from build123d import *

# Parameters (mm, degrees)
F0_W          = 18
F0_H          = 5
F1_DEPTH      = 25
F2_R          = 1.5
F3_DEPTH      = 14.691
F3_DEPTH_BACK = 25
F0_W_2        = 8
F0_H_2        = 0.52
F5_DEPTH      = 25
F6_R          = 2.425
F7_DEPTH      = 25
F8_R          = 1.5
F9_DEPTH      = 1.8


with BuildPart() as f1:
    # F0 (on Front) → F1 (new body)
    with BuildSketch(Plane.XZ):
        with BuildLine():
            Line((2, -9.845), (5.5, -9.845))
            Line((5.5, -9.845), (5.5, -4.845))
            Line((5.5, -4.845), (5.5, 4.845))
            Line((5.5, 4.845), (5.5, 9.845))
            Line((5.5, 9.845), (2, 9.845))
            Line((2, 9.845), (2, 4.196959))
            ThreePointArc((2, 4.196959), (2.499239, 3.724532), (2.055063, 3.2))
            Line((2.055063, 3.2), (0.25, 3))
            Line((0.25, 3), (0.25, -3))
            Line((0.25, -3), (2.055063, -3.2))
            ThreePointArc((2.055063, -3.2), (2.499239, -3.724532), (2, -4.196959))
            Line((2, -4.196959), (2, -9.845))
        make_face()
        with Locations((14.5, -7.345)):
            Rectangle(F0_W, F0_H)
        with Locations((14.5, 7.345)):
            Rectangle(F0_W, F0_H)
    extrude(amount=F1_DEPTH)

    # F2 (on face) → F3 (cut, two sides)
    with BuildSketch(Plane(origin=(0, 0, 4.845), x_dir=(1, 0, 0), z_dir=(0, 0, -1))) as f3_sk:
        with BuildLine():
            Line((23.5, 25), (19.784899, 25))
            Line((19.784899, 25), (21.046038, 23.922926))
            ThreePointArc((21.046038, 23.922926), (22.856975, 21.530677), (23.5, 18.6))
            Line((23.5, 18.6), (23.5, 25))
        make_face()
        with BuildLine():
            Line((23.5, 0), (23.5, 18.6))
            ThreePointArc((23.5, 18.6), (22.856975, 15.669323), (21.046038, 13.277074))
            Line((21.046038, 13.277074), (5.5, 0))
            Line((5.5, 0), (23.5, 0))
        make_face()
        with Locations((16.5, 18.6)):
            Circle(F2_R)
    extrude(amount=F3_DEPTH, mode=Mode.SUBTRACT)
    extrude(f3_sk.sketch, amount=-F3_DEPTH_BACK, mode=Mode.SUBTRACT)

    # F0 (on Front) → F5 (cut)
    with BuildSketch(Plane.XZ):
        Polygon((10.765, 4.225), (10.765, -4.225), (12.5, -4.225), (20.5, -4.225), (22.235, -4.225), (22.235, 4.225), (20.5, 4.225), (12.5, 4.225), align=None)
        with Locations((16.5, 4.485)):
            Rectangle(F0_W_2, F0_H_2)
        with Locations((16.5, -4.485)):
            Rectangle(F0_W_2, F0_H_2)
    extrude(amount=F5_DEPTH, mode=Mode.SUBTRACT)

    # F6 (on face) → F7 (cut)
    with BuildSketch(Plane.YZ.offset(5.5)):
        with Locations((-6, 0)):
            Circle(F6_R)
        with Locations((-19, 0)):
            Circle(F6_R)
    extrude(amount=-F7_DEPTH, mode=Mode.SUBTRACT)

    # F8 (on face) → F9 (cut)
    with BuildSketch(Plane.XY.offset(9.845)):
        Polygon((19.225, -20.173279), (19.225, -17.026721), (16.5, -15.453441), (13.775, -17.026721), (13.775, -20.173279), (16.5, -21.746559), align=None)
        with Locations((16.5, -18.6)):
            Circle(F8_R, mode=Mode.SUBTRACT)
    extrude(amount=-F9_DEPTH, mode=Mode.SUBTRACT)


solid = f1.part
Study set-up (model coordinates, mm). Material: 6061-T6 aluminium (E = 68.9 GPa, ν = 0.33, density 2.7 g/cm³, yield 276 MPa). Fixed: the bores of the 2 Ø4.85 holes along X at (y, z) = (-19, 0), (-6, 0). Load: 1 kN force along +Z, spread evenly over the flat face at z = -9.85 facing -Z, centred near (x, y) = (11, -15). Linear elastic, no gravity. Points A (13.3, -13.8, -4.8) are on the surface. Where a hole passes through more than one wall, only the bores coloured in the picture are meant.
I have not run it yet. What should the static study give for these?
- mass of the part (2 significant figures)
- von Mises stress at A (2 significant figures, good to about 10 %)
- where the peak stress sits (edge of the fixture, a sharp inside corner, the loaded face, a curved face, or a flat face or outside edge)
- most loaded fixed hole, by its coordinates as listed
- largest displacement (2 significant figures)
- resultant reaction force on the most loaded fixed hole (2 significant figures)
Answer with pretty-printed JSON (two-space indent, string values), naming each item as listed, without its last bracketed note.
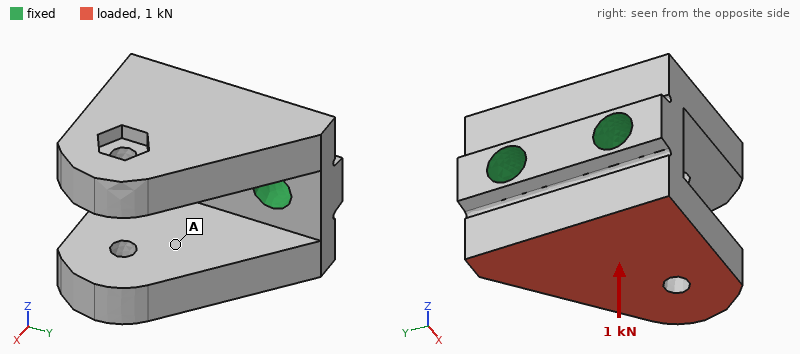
{
  "mass of the part": "13 g",
  "von Mises stress at A": "27 MPa",
  "where the peak stress sits": "a curved face",
  "most loaded fixed hole, by its coordinates as listed": "(-19, 0)",
  "largest displacement": "0.17 mm",
  "resultant reaction force on the most loaded fixed hole": "650 N"
}
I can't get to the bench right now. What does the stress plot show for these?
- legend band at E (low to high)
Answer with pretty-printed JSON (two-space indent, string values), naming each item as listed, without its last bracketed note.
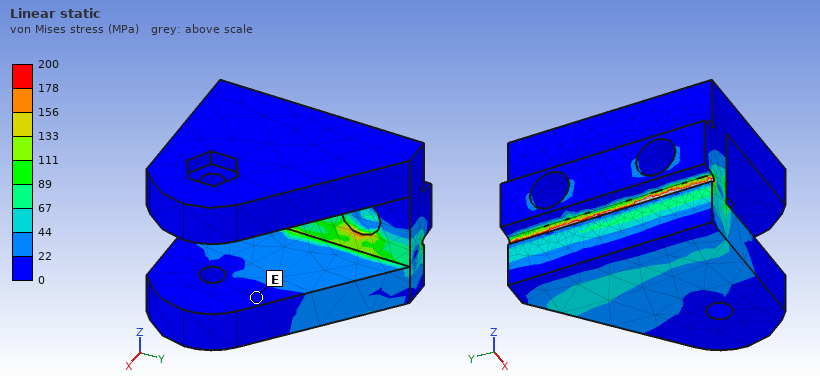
{
  "legend band at E": "0 to 22 MPa"
}
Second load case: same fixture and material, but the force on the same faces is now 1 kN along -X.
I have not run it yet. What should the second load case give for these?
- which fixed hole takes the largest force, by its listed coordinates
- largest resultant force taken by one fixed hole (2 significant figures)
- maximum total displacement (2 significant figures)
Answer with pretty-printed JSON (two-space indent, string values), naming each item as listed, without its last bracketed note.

{
  "which fixed hole takes the largest force, by its listed coordinates": "(-19, 0)",
  "largest resultant force taken by one fixed hole": "640 N",
  "maximum total displacement": "0.13 mm"
}
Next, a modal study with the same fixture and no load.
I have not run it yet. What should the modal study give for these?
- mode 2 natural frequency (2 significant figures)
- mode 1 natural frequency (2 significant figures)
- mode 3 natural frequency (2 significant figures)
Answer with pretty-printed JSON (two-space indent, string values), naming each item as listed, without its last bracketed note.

{
  "mode 2 natural frequency": "7000 Hz",
  "mode 1 natural frequency": "6800 Hz",
  "mode 3 natural frequency": "17 kHz"
}
